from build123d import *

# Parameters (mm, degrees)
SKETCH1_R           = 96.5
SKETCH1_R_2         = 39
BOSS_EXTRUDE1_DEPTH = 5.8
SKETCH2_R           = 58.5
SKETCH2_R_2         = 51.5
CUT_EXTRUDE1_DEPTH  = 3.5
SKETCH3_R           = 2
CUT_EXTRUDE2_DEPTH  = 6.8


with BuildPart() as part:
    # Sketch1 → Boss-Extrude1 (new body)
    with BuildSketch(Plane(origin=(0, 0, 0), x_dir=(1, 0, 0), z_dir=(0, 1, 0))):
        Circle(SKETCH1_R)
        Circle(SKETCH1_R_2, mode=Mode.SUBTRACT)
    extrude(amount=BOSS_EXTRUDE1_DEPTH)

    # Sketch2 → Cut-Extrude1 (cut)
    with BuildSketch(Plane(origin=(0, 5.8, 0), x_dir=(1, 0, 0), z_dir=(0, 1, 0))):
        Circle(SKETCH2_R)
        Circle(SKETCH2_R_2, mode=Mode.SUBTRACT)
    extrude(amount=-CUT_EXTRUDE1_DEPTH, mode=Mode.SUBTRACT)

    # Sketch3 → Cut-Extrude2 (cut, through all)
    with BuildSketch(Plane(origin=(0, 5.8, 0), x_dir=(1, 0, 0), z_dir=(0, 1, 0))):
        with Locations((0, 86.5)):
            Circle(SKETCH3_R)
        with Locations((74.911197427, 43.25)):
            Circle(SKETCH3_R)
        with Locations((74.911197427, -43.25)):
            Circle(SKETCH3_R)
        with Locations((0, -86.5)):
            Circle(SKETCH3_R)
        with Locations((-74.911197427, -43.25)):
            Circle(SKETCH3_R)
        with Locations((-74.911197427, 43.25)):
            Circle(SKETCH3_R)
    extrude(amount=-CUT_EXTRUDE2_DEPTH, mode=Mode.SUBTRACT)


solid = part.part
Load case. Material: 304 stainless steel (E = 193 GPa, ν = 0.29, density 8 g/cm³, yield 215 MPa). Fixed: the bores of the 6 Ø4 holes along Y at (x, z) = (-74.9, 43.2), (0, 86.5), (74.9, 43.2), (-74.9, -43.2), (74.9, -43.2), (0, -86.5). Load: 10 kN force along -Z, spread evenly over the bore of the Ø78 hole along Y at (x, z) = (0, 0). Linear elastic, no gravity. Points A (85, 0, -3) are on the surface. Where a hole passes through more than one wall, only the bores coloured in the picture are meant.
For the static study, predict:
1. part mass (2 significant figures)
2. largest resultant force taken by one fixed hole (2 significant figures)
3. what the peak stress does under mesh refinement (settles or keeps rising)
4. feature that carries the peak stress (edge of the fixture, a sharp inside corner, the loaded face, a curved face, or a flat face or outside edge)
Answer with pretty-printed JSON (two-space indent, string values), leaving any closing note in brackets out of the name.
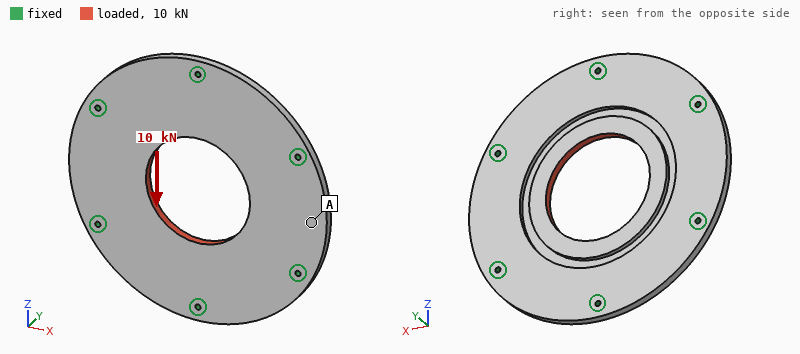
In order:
{
  "part mass": "1.1 kg",
  "largest resultant force taken by one fixed hole": "2.1 kN",
  "what the peak stress does under mesh refinement": "keeps rising",
  "feature that carries the peak stress": "edge of the fixture"
}
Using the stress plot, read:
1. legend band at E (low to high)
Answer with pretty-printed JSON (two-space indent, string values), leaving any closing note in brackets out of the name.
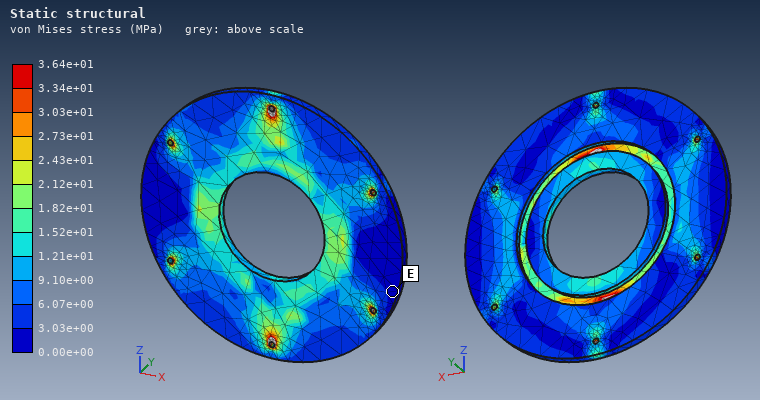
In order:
{
  "legend band at E": "0.00e+00 to 3.03e+00 MPa"
}
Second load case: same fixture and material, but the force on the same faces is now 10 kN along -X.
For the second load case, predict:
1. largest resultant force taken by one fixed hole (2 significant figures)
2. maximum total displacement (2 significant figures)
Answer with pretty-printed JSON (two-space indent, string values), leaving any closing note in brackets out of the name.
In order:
{
  "largest resultant force taken by one fixed hole": "1.9 kN",
  "maximum total displacement": "10.0 µm"
}
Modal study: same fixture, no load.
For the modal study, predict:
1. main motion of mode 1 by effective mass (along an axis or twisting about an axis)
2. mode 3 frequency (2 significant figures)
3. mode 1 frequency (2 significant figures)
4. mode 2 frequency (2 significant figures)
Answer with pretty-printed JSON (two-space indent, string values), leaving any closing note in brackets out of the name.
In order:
{
  "main motion of mode 1 by effective mass": "along Y",
  "mode 3 frequency": "2600 Hz",
  "mode 1 frequency": "1900 Hz",
  "mode 2 frequency": "2600 Hz"
}
